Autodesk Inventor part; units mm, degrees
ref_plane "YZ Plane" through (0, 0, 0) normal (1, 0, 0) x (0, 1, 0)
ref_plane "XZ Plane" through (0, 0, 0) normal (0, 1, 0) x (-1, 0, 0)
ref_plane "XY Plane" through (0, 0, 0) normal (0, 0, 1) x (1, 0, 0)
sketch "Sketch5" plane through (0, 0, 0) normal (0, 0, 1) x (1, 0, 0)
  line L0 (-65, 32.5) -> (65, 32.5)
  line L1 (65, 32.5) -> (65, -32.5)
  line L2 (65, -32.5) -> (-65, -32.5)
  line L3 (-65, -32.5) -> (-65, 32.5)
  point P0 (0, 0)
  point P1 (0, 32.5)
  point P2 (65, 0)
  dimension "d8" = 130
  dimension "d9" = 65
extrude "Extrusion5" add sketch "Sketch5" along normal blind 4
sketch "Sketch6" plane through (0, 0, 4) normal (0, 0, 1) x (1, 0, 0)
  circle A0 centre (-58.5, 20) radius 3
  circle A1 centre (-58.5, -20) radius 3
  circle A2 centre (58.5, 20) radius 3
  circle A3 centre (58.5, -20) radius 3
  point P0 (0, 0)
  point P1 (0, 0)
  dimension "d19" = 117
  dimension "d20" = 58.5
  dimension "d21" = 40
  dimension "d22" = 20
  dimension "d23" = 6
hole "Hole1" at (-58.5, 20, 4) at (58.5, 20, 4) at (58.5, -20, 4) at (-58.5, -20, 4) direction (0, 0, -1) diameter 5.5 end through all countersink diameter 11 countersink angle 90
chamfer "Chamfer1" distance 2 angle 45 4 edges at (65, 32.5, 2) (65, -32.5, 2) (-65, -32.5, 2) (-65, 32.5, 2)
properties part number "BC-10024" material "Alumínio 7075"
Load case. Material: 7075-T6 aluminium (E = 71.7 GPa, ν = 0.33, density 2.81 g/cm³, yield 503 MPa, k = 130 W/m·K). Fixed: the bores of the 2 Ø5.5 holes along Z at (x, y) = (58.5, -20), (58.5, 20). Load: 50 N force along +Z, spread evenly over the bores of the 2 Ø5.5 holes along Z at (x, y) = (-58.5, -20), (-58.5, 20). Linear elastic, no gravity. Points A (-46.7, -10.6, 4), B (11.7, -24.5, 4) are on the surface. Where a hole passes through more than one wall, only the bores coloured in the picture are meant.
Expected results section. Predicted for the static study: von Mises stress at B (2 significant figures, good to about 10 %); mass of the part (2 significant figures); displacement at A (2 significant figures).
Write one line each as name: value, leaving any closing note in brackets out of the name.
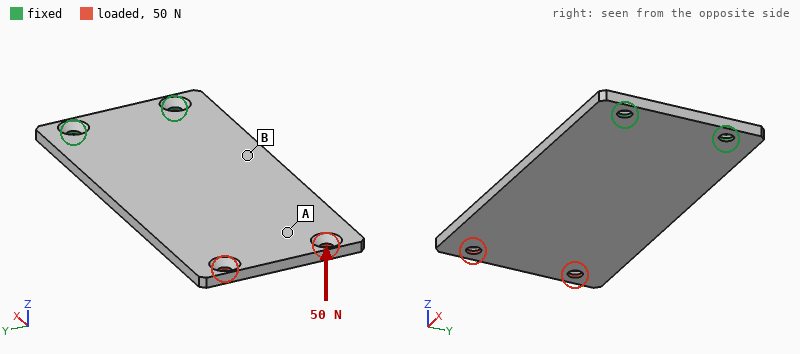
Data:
von Mises stress at B: 20 MPa
mass of the part: 93 g
displacement at A: 1.2 mm
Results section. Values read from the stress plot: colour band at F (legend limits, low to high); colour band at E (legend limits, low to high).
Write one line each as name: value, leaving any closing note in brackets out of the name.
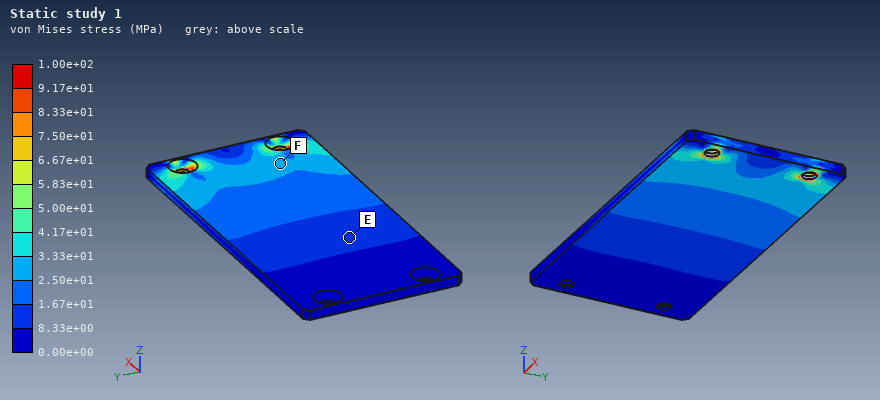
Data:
colour band at F: 2.50e+01 to 3.33e+01 MPa
colour band at E: 8.33e+00 to 1.67e+01 MPa
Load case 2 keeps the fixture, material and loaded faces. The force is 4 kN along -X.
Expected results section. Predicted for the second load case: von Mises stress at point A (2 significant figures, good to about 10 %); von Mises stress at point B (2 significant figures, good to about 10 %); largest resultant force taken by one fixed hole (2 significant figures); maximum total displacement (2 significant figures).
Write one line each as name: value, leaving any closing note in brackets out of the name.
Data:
von Mises stress at point A: 17 MPa
von Mises stress at point B: 16 MPa
largest resultant force taken by one fixed hole: 2.0 kN
maximum total displacement: 1.6 mm
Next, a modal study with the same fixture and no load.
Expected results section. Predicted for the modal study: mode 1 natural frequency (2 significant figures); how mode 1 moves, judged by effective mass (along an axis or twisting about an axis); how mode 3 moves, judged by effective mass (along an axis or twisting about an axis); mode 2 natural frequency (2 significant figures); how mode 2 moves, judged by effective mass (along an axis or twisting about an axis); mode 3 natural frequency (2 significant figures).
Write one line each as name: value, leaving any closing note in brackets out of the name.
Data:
mode 1 natural frequency: 180 Hz
how mode 1 moves, judged by effective mass: along Z
how mode 3 moves, judged by effective mass: along Z
mode 2 natural frequency: 840 Hz
how mode 2 moves, judged by effective mass: twisting about X
mode 3 natural frequency: 1200 Hz
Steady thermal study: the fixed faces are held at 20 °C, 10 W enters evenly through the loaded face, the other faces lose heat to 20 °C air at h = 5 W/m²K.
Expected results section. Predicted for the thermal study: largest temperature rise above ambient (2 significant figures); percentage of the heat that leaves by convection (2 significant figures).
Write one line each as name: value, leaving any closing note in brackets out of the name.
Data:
largest temperature rise above ambient: 37 K
percentage of the heat that leaves by convection: 16 %
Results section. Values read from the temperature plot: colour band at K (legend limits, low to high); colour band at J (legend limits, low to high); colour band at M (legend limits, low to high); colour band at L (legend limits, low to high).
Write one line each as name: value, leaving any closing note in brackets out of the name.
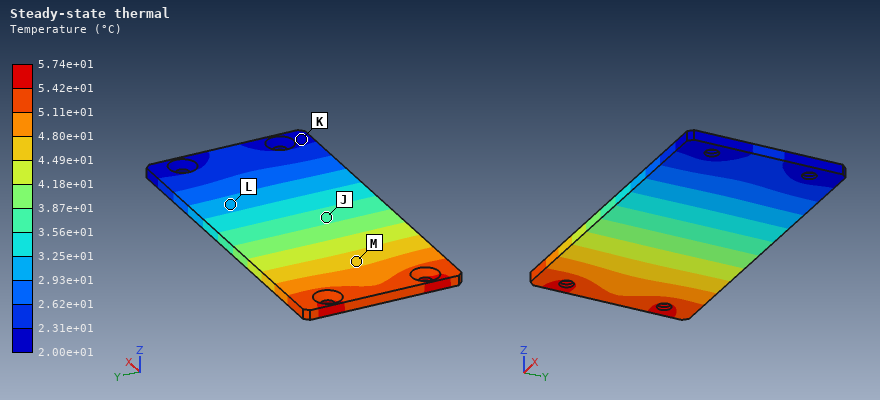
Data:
colour band at K: 2.00e+01 to 2.31e+01 °C
colour band at J: 3.56e+01 to 3.87e+01 °C
colour band at M: 4.49e+01 to 4.80e+01 °C
colour band at L: 2.93e+01 to 3.25e+01 °C
